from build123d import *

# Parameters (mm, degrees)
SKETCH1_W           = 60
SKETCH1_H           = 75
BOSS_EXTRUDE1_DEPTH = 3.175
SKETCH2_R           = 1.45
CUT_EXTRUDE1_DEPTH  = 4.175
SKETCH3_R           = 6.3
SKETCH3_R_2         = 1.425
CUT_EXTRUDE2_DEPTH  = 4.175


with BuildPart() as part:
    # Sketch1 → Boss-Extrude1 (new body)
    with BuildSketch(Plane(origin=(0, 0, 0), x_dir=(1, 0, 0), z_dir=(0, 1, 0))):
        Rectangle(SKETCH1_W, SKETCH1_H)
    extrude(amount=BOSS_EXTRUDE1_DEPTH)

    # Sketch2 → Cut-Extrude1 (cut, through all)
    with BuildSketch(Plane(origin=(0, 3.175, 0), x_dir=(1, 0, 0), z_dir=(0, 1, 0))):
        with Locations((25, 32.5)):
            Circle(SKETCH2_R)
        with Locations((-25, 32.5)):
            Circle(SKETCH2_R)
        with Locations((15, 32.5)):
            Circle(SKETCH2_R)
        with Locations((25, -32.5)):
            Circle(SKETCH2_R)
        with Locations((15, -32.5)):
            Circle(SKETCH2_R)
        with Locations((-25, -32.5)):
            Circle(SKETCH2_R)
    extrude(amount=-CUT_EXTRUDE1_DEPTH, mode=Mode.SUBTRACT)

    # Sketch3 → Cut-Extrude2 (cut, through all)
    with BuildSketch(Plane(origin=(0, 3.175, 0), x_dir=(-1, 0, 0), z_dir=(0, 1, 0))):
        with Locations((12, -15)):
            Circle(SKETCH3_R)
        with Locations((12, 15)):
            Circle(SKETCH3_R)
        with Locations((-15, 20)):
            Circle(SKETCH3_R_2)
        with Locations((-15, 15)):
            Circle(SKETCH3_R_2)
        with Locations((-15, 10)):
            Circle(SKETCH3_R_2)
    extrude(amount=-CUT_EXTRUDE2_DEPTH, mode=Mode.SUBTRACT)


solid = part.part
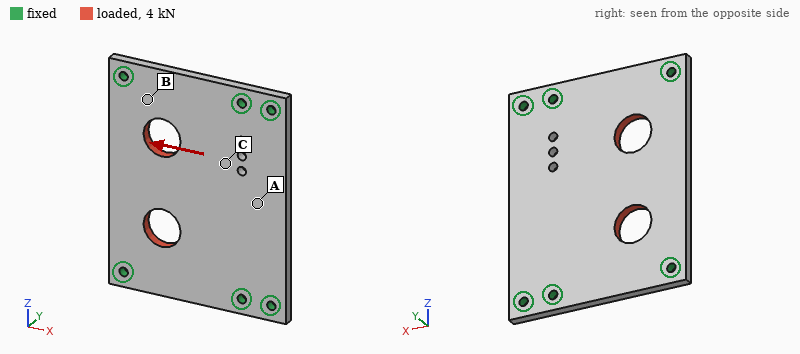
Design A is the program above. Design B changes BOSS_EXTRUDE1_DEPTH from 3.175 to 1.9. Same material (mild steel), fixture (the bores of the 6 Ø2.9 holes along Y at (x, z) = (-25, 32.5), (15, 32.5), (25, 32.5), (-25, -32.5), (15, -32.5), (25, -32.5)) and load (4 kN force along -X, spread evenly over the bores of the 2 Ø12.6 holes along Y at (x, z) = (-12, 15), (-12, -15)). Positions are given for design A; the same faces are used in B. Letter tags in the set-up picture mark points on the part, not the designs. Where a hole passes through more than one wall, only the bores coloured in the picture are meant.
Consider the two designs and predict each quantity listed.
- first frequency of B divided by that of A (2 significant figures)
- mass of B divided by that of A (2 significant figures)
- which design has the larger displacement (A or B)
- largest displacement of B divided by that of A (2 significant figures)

0.62
0.60
B
1.7
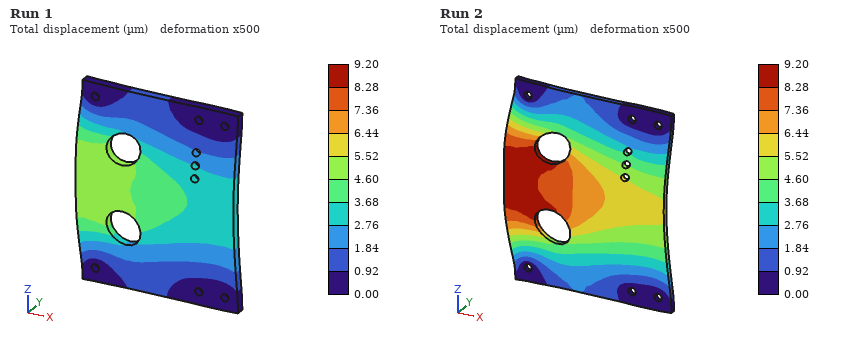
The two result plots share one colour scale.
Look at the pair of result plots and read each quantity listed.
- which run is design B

Run 2
